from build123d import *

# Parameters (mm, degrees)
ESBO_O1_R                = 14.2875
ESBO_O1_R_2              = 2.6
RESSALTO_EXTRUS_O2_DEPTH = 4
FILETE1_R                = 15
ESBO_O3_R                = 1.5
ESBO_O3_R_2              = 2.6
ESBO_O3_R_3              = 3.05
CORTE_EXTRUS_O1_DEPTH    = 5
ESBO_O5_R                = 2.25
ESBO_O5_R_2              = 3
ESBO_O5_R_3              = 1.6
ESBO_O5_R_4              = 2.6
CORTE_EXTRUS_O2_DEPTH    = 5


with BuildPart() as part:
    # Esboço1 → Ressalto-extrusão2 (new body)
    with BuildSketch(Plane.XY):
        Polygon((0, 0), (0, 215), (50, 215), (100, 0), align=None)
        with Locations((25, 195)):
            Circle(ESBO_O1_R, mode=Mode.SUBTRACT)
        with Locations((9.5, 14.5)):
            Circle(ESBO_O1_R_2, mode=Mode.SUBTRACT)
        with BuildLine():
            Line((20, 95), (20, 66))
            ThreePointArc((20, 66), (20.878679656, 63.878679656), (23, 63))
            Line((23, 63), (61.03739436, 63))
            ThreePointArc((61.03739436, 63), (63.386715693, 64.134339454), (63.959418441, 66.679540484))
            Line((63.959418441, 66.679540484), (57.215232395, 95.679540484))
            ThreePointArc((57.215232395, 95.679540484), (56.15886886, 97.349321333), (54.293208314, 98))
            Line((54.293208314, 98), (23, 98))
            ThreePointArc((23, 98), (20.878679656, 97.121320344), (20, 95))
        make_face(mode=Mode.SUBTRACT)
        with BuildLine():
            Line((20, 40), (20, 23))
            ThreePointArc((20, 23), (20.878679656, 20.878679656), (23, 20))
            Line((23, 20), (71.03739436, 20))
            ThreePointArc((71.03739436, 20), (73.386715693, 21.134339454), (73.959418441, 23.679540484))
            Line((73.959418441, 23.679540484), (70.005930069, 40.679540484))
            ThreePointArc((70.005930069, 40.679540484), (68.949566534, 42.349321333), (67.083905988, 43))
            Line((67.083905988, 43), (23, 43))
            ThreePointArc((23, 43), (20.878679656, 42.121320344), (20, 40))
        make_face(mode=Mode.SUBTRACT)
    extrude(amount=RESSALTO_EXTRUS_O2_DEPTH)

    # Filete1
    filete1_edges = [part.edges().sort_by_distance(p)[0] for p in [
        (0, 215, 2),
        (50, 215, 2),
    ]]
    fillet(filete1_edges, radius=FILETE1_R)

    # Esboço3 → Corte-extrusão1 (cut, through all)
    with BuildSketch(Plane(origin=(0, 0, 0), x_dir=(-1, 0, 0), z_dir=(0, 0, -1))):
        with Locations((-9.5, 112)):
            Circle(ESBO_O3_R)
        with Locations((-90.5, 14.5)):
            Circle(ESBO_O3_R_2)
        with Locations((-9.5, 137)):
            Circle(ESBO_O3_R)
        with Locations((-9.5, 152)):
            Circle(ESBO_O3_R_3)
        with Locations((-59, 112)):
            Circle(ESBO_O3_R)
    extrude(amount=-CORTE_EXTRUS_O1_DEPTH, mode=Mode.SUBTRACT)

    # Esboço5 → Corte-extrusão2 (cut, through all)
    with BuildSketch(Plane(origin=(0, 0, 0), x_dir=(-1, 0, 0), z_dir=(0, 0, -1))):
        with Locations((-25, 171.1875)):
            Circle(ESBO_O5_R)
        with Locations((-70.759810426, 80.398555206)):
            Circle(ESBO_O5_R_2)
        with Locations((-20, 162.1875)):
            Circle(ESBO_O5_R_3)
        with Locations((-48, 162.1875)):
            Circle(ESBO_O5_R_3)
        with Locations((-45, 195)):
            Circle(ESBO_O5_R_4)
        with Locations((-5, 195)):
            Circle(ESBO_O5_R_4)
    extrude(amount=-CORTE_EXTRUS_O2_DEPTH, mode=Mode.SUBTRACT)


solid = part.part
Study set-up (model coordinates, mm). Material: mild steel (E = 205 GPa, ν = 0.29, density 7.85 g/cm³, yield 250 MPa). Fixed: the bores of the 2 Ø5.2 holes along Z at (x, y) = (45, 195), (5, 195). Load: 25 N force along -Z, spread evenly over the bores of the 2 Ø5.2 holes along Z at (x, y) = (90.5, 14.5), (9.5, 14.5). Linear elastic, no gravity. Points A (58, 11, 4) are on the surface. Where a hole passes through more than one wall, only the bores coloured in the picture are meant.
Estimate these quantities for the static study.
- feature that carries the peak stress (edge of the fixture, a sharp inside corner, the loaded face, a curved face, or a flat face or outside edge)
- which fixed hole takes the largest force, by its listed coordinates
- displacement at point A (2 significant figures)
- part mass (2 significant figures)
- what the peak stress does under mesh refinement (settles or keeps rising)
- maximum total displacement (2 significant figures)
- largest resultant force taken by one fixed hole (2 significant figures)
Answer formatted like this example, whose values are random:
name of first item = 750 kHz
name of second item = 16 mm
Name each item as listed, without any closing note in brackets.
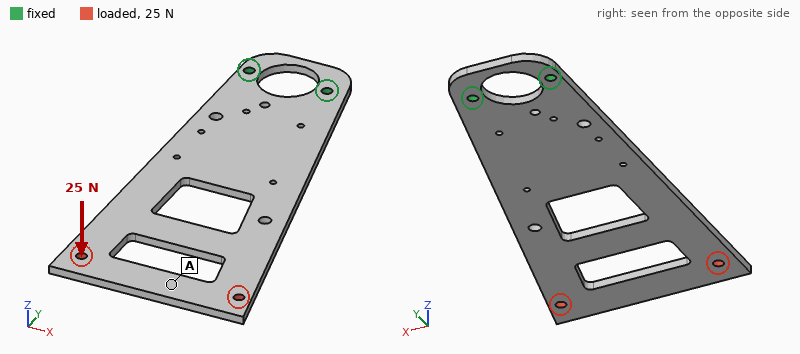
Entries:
feature that carries the peak stress = edge of the fixture
which fixed hole takes the largest force, by its listed coordinates = (45, 195)
displacement at point A = 0.96 mm
part mass = 400 g
what the peak stress does under mesh refinement = keeps rising
maximum total displacement = 1.1 mm
largest resultant force taken by one fixed hole = 27 N
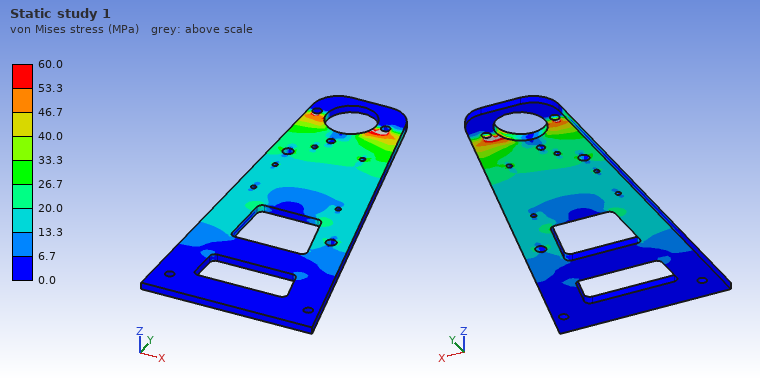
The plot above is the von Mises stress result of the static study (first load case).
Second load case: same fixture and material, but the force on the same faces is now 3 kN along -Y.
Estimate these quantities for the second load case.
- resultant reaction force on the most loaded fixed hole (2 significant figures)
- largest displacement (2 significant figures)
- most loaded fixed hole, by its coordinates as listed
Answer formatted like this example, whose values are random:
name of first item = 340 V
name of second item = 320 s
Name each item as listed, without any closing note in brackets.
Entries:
resultant reaction force on the most loaded fixed hole = 3.3 kN
largest displacement = 92 µm
most loaded fixed hole, by its coordinates as listed = (45, 195)
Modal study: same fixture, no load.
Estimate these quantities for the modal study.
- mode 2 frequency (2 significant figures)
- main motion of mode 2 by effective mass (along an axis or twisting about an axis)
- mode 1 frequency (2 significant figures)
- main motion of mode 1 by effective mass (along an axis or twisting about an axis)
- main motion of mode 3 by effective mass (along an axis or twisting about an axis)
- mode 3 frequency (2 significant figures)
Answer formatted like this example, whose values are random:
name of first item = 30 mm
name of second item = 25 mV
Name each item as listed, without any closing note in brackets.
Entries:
mode 2 frequency = 320 Hz
main motion of mode 2 by effective mass = twisting about Y
mode 1 frequency = 72 Hz
main motion of mode 1 by effective mass = along Z
main motion of mode 3 by effective mass = along Z
mode 3 frequency = 440 Hz
